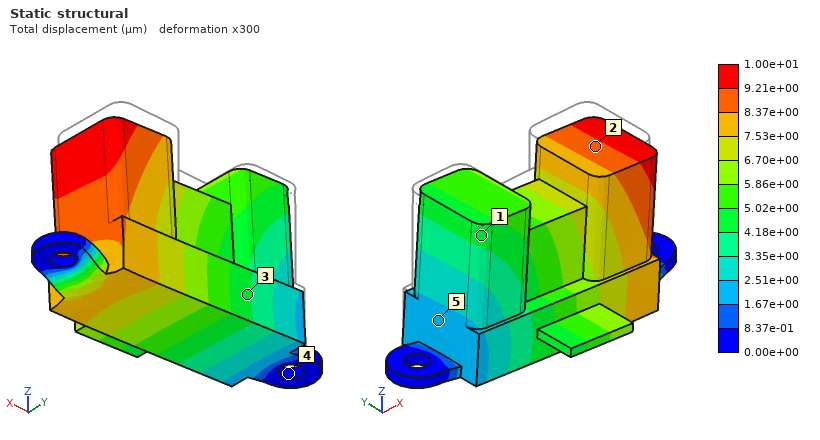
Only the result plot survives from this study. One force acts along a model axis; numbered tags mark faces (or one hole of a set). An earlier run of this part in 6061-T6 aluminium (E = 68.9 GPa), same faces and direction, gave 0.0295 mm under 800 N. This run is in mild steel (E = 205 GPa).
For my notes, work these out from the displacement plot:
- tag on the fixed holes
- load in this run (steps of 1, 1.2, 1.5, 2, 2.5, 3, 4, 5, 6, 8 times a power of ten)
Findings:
4
800 N
